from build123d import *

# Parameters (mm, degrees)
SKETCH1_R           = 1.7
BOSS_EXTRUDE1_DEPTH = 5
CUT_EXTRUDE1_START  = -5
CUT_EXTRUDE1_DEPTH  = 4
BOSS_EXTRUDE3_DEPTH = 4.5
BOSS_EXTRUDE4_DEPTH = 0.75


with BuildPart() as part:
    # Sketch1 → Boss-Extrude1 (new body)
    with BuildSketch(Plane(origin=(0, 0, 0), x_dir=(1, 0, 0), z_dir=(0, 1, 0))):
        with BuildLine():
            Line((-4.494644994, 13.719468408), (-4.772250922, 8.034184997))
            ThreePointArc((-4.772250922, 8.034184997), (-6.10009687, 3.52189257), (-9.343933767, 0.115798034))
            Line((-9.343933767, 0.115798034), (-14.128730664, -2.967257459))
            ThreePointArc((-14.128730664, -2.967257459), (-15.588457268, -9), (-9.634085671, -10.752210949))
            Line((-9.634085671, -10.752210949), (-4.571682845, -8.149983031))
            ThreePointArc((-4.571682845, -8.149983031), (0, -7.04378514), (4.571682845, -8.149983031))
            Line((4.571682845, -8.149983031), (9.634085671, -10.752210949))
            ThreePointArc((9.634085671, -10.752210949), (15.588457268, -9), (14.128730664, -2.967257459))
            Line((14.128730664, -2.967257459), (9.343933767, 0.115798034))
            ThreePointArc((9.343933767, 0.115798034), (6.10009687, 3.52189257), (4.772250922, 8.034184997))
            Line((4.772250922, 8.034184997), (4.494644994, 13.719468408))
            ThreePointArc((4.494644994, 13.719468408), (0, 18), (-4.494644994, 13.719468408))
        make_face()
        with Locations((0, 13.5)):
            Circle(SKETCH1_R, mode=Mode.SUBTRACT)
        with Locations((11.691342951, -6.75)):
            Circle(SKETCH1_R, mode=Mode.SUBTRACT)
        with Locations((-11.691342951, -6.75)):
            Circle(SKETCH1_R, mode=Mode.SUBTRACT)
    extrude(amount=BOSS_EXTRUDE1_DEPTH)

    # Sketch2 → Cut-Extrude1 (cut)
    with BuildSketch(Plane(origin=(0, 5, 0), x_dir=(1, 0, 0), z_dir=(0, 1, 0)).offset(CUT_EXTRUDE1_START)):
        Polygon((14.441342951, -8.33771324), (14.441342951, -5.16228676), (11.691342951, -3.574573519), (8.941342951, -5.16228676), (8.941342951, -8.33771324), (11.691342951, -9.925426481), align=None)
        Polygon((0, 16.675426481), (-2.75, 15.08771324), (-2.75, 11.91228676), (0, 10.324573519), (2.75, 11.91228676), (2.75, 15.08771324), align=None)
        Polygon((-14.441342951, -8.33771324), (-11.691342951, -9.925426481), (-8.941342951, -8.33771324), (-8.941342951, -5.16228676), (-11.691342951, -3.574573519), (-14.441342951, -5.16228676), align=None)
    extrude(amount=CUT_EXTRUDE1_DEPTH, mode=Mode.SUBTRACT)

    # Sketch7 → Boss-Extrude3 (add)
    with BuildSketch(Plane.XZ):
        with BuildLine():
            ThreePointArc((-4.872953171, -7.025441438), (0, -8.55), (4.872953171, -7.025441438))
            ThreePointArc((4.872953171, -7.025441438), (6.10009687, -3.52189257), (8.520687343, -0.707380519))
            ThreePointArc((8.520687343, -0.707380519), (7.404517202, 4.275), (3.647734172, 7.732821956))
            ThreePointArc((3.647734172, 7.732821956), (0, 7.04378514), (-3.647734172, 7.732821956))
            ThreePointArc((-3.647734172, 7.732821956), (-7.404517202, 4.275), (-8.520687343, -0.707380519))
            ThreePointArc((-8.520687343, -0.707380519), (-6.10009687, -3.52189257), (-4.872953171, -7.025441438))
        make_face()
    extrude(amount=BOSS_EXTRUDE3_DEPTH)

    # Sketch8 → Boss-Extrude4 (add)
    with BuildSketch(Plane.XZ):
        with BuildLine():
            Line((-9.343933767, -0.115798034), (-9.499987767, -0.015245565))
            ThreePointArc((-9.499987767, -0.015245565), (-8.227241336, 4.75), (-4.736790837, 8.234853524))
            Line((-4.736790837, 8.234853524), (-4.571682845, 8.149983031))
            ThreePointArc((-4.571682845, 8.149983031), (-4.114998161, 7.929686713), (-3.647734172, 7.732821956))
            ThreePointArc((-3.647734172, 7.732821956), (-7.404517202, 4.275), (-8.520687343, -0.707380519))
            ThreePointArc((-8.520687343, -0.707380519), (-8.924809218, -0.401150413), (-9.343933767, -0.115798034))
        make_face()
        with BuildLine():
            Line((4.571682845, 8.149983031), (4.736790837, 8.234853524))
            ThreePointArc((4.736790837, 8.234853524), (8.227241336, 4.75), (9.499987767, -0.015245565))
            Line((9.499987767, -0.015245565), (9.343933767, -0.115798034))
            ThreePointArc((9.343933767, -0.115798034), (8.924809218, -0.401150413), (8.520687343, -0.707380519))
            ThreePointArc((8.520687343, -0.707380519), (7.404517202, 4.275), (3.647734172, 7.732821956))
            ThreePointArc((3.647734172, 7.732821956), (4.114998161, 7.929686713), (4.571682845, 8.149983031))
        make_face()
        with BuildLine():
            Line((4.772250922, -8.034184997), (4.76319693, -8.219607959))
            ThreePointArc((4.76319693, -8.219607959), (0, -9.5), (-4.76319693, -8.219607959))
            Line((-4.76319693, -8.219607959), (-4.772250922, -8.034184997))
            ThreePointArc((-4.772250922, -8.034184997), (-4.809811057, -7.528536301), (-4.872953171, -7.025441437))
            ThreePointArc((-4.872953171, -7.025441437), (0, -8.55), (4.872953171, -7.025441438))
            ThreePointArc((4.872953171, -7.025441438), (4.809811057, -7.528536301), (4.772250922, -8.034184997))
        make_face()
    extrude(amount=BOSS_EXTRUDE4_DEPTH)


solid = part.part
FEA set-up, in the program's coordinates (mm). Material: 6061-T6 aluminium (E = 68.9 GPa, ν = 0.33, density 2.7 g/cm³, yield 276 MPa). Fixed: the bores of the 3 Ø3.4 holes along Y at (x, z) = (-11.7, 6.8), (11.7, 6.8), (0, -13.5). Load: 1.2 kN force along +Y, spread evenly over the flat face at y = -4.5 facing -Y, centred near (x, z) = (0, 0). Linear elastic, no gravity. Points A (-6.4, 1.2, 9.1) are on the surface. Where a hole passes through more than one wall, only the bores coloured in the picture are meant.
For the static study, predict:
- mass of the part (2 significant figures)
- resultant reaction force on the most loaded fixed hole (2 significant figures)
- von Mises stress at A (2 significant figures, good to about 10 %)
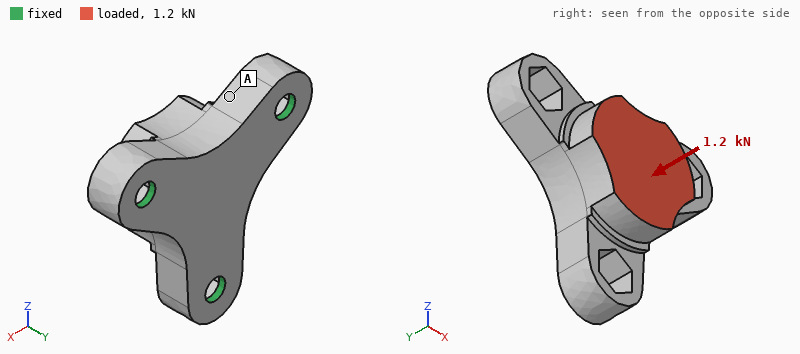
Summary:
7.8 g
510 N
22 MPa
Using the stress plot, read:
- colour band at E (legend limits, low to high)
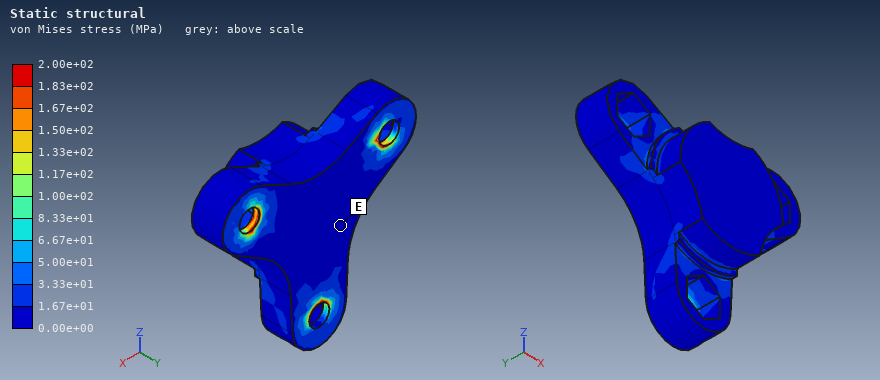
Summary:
0.00e+00 to 1.67e+01 MPa
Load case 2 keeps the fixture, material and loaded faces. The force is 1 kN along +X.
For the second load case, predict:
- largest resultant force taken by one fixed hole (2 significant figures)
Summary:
640 N
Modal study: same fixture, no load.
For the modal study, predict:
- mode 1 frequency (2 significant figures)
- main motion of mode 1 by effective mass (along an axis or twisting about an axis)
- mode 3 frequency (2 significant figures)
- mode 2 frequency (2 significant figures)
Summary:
23 kHz
along Y
29 kHz
29 kHz
